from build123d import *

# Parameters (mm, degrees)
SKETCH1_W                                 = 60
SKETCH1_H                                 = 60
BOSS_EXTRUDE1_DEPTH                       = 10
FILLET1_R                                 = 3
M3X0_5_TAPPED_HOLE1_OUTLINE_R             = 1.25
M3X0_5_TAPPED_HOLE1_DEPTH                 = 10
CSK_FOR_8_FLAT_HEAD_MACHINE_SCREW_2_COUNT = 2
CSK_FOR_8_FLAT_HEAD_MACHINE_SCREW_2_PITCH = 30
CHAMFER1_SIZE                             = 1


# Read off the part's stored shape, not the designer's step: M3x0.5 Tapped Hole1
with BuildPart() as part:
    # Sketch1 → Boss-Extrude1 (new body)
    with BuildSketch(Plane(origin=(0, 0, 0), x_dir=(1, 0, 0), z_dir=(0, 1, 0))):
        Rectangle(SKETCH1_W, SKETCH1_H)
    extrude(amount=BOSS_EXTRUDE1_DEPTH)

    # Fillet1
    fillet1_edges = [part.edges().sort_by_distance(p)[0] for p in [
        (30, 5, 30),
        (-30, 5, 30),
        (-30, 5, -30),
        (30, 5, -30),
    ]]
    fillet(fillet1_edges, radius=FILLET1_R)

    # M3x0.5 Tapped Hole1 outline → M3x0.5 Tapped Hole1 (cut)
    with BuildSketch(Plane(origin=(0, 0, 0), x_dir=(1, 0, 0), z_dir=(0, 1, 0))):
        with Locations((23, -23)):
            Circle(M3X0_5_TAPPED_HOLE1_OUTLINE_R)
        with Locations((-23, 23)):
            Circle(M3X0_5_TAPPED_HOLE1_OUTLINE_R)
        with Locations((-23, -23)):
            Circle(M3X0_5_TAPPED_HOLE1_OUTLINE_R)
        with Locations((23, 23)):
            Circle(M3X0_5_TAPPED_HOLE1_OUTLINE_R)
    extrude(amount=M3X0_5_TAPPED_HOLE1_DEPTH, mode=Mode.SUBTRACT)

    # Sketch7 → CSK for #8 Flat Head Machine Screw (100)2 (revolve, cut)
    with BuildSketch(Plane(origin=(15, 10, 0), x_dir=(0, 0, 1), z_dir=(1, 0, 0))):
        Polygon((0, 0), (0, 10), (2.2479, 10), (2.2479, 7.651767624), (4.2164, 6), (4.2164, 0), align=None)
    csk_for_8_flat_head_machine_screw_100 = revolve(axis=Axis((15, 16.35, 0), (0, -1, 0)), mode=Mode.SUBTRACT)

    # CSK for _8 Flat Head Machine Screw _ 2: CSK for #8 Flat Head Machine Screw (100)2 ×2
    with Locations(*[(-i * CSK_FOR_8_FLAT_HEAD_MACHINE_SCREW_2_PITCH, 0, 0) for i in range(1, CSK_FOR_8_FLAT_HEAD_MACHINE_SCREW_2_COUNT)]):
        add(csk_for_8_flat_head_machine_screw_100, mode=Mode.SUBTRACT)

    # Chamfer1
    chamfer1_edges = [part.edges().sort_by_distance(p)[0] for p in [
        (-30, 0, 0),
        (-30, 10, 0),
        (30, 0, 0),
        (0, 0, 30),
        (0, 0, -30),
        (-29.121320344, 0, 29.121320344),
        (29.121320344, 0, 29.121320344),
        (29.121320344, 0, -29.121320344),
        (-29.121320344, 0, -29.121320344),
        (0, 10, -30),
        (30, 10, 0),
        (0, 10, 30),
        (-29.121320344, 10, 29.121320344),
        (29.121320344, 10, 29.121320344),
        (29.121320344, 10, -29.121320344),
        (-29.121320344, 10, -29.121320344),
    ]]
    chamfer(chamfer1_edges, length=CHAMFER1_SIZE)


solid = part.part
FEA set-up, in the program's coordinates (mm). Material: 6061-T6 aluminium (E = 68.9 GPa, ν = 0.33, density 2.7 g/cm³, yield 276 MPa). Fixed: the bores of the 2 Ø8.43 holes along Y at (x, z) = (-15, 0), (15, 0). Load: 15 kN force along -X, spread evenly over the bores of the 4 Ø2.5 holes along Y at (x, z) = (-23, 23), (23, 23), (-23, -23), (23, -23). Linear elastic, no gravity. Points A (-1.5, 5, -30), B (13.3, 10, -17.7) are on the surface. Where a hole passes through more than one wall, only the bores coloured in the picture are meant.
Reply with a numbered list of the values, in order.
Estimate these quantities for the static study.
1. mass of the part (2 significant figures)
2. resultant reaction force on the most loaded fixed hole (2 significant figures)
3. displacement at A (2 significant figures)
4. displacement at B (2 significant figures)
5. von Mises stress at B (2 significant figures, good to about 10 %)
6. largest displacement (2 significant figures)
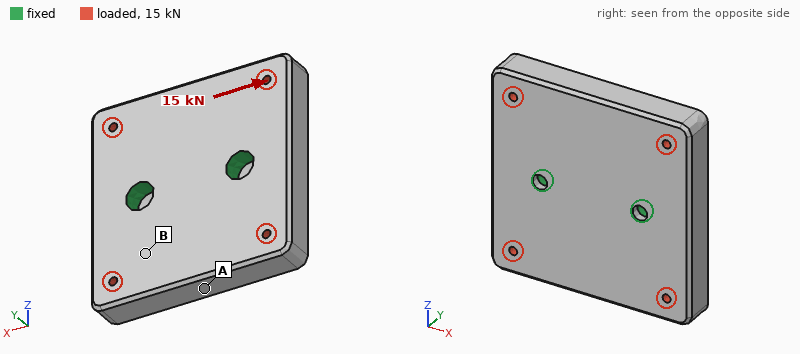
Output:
1. 94 g
2. 7.5 kN
3. 15 µm
4. 11 µm
5. 25 MPa
6. 21 µm
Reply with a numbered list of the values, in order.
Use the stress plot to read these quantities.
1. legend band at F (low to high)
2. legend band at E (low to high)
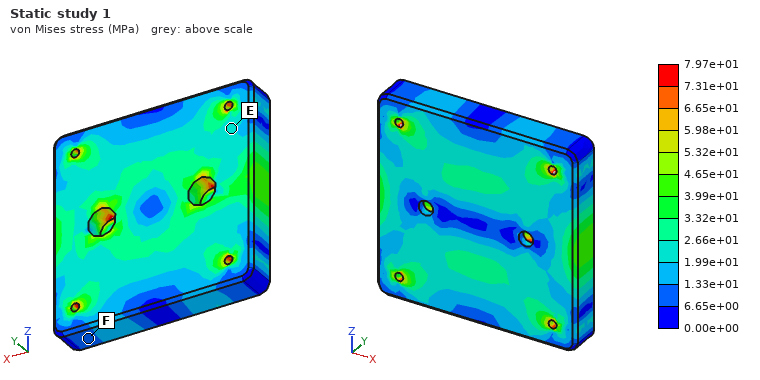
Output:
1. 6.65e+00 to 1.33e+01 MPa
2. 1.99e+01 to 2.66e+01 MPa
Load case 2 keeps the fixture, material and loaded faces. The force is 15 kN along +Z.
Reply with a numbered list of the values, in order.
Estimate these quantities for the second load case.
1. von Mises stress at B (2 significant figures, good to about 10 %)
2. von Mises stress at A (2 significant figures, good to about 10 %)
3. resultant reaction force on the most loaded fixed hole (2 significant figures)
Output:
1. 15 MPa
2. 19 MPa
3. 7.5 kN
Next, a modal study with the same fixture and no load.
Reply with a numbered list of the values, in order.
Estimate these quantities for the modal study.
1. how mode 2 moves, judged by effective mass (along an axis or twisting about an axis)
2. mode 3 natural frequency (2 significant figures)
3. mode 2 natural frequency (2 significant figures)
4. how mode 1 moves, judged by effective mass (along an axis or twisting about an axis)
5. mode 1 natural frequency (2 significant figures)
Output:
1. along Y
2. 11 kHz
3. 9200 Hz
4. twisting about X
5. 6700 Hz
